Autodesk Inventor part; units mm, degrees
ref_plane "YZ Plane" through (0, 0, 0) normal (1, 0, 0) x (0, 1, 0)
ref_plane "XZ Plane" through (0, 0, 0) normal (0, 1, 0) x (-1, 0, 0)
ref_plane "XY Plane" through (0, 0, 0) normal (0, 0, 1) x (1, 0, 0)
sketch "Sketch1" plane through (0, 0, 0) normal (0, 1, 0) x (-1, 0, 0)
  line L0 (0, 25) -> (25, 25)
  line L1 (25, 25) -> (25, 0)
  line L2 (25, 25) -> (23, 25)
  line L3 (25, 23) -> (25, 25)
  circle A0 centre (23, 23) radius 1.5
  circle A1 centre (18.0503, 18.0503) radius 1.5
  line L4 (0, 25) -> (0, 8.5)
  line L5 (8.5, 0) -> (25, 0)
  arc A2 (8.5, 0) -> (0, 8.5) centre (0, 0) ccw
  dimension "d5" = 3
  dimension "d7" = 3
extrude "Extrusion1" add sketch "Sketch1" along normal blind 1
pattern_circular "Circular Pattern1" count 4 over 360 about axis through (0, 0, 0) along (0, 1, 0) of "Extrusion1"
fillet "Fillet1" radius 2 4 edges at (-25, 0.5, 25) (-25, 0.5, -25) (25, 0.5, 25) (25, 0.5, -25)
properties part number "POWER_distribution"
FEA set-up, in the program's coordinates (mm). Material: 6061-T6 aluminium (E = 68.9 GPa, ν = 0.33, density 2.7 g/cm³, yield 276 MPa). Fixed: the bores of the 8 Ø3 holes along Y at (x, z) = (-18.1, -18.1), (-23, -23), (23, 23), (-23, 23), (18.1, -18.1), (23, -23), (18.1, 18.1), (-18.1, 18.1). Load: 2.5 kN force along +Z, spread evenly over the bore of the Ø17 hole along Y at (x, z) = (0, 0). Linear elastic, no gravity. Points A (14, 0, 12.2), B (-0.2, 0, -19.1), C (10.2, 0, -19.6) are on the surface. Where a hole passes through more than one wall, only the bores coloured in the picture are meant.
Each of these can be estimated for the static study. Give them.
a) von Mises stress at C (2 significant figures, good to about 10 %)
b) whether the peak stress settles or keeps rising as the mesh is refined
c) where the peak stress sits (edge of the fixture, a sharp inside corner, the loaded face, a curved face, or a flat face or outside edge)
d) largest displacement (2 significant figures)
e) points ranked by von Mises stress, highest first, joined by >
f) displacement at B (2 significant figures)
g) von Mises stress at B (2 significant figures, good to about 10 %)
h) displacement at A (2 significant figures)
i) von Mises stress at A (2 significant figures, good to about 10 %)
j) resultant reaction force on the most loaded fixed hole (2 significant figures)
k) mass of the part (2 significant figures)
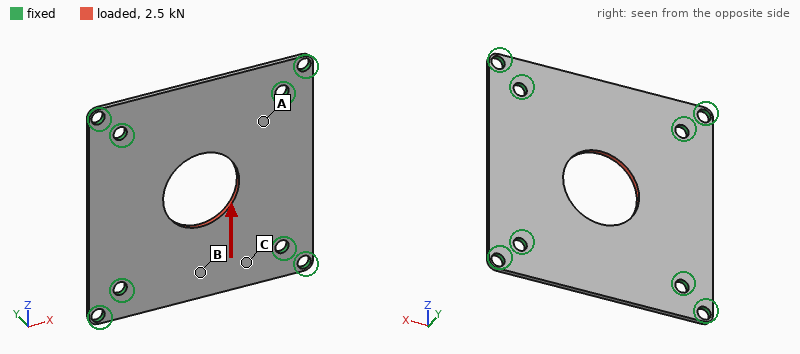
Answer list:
35 MPa
keeps rising
edge of the fixture
21 µm
A > C > B
17 µm
17 MPa
7.0 µm
56 MPa
570 N
6.0 g
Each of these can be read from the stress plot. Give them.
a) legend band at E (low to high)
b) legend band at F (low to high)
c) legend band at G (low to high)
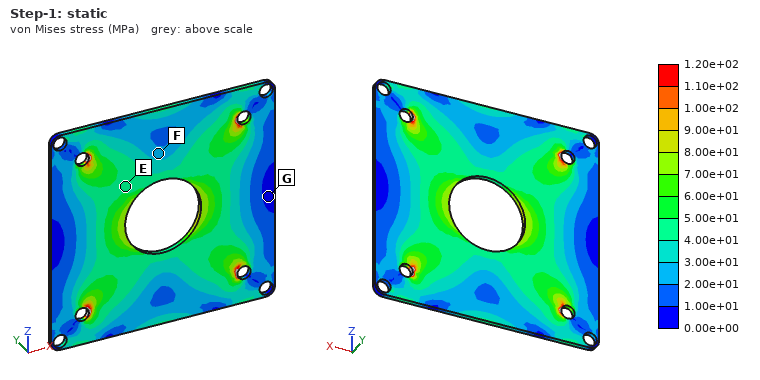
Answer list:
4.00e+01 to 5.00e+01 MPa
2.00e+01 to 3.00e+01 MPa
0.00e+00 to 1.00e+01 MPa
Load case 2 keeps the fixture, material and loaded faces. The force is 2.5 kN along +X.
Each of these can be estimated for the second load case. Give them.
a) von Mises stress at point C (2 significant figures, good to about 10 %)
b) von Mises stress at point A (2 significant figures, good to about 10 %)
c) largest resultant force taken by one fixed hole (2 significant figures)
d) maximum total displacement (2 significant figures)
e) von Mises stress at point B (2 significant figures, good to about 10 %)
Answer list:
29 MPa
55 MPa
570 N
21 µm
21 MPa
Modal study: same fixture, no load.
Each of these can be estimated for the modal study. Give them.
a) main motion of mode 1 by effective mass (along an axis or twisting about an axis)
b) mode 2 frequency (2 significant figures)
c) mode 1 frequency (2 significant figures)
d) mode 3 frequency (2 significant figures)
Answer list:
along Y
4500 Hz
3400 Hz
4500 Hz
